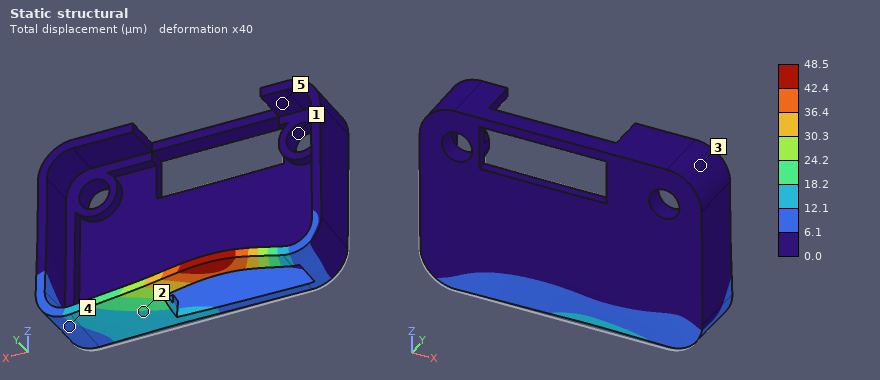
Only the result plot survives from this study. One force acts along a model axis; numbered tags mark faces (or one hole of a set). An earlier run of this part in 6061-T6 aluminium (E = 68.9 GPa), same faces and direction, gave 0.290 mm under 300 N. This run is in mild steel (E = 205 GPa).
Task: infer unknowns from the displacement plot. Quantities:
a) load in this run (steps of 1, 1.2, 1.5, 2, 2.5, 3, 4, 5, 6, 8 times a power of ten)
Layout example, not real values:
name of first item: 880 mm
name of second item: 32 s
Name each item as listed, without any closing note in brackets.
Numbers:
load in this run: 150 N
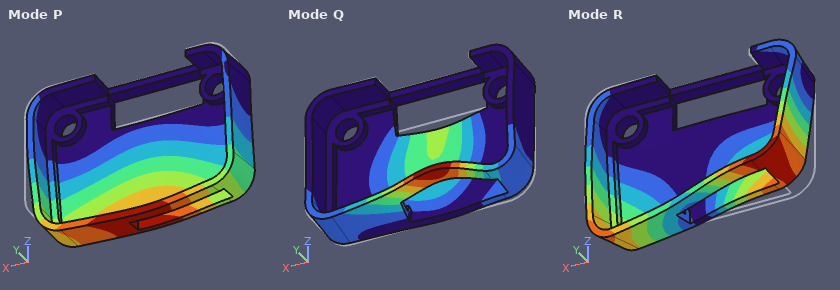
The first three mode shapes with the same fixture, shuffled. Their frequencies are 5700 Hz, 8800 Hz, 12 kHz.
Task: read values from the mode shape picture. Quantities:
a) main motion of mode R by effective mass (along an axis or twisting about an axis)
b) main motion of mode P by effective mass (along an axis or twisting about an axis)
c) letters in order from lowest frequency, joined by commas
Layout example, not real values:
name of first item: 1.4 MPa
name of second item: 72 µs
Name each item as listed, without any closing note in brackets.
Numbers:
main motion of mode R by effective mass: twisting about Z
main motion of mode P by effective mass: along Y
letters in order from lowest frequency, joined by commas: P, R, Q
